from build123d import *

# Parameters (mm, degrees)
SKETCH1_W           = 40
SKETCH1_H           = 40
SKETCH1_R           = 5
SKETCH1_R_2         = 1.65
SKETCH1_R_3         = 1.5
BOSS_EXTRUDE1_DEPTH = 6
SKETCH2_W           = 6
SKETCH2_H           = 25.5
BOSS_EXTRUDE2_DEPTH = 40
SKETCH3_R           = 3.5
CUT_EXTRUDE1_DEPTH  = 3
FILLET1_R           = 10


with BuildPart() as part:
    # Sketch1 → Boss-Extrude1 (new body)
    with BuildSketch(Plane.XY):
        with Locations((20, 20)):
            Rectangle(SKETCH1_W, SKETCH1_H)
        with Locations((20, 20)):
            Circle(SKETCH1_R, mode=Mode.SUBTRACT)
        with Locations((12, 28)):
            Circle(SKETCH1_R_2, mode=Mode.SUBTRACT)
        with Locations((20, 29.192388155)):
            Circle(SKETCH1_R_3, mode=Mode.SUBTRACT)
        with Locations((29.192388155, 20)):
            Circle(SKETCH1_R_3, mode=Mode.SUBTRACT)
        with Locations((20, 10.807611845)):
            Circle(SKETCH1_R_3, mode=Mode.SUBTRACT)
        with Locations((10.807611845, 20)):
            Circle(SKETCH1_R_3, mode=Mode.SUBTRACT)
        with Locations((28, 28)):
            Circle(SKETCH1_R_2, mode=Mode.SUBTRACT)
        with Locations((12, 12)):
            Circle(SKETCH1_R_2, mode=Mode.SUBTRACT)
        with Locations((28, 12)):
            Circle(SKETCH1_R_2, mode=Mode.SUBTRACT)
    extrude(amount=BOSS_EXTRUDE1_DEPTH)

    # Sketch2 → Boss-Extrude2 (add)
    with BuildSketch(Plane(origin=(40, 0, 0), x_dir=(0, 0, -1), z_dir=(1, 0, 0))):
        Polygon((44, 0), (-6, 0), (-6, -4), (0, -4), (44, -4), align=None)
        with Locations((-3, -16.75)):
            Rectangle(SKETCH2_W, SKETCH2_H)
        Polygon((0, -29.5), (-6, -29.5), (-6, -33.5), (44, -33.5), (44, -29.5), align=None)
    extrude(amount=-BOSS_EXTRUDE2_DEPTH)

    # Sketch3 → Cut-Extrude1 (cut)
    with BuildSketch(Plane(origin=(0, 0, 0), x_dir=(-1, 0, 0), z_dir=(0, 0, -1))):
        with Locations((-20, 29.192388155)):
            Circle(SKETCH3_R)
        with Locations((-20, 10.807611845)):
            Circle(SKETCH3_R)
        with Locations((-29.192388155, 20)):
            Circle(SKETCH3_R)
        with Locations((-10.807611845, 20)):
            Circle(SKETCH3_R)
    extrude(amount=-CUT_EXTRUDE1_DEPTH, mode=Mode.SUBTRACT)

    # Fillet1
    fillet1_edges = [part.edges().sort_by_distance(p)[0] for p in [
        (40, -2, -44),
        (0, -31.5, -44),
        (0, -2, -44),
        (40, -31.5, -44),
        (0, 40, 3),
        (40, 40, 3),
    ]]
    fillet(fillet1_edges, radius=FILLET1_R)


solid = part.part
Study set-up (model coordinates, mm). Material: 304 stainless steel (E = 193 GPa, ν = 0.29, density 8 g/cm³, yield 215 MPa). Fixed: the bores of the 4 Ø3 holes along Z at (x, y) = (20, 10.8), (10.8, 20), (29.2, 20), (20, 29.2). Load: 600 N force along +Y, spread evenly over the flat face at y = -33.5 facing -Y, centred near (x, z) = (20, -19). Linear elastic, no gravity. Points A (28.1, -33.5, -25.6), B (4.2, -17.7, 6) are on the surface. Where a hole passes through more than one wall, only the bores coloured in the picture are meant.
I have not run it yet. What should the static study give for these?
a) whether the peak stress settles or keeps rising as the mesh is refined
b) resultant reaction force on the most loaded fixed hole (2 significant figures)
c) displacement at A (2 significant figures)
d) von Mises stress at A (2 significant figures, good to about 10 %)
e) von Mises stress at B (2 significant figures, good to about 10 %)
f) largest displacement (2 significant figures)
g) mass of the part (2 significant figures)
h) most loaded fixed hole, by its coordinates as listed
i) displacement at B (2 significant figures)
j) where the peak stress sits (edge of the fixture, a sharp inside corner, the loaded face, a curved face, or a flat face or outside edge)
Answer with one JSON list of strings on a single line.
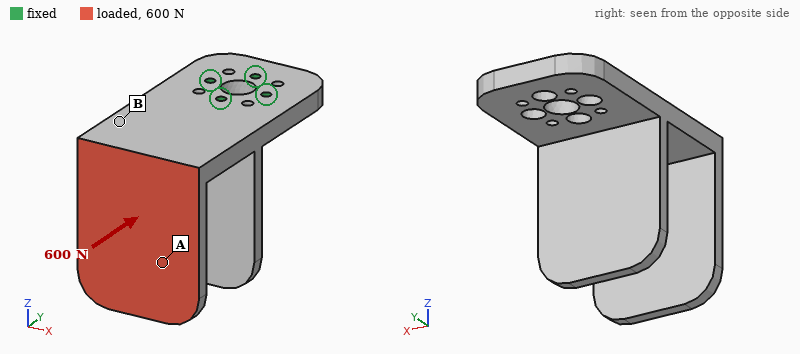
["keeps rising", "1.0 kN", "0.23 mm", "17 MPa", "51 MPa", "0.37 mm", "240 g", "(20, 10.8)", "0.058 mm", "edge of the fixture"]
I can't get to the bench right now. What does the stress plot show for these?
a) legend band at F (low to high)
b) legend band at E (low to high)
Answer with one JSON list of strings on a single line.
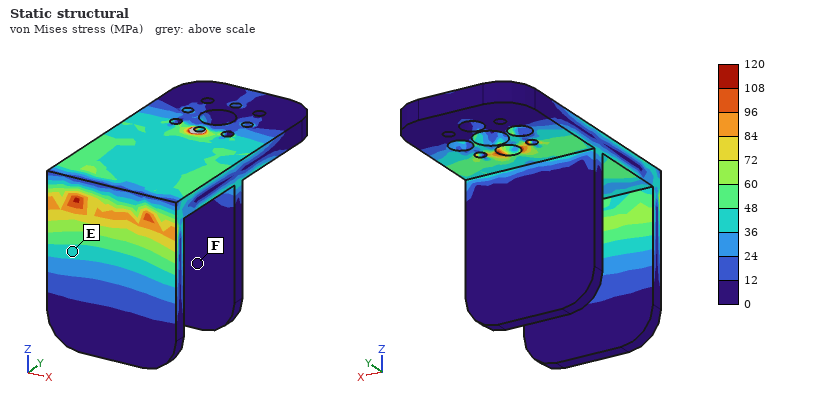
["0 to 12 MPa", "36 to 48 MPa"]
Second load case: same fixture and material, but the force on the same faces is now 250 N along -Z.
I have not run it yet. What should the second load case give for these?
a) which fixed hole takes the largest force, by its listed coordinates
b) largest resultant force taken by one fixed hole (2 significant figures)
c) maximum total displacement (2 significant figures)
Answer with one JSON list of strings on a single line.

["(20, 10.8)", "1.1 kN", "0.14 mm"]
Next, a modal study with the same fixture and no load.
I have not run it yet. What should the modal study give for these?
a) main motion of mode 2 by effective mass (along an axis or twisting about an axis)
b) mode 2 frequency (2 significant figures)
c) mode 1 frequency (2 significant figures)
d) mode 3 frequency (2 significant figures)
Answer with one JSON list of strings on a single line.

["along X", "1300 Hz", "760 Hz", "1400 Hz"]
